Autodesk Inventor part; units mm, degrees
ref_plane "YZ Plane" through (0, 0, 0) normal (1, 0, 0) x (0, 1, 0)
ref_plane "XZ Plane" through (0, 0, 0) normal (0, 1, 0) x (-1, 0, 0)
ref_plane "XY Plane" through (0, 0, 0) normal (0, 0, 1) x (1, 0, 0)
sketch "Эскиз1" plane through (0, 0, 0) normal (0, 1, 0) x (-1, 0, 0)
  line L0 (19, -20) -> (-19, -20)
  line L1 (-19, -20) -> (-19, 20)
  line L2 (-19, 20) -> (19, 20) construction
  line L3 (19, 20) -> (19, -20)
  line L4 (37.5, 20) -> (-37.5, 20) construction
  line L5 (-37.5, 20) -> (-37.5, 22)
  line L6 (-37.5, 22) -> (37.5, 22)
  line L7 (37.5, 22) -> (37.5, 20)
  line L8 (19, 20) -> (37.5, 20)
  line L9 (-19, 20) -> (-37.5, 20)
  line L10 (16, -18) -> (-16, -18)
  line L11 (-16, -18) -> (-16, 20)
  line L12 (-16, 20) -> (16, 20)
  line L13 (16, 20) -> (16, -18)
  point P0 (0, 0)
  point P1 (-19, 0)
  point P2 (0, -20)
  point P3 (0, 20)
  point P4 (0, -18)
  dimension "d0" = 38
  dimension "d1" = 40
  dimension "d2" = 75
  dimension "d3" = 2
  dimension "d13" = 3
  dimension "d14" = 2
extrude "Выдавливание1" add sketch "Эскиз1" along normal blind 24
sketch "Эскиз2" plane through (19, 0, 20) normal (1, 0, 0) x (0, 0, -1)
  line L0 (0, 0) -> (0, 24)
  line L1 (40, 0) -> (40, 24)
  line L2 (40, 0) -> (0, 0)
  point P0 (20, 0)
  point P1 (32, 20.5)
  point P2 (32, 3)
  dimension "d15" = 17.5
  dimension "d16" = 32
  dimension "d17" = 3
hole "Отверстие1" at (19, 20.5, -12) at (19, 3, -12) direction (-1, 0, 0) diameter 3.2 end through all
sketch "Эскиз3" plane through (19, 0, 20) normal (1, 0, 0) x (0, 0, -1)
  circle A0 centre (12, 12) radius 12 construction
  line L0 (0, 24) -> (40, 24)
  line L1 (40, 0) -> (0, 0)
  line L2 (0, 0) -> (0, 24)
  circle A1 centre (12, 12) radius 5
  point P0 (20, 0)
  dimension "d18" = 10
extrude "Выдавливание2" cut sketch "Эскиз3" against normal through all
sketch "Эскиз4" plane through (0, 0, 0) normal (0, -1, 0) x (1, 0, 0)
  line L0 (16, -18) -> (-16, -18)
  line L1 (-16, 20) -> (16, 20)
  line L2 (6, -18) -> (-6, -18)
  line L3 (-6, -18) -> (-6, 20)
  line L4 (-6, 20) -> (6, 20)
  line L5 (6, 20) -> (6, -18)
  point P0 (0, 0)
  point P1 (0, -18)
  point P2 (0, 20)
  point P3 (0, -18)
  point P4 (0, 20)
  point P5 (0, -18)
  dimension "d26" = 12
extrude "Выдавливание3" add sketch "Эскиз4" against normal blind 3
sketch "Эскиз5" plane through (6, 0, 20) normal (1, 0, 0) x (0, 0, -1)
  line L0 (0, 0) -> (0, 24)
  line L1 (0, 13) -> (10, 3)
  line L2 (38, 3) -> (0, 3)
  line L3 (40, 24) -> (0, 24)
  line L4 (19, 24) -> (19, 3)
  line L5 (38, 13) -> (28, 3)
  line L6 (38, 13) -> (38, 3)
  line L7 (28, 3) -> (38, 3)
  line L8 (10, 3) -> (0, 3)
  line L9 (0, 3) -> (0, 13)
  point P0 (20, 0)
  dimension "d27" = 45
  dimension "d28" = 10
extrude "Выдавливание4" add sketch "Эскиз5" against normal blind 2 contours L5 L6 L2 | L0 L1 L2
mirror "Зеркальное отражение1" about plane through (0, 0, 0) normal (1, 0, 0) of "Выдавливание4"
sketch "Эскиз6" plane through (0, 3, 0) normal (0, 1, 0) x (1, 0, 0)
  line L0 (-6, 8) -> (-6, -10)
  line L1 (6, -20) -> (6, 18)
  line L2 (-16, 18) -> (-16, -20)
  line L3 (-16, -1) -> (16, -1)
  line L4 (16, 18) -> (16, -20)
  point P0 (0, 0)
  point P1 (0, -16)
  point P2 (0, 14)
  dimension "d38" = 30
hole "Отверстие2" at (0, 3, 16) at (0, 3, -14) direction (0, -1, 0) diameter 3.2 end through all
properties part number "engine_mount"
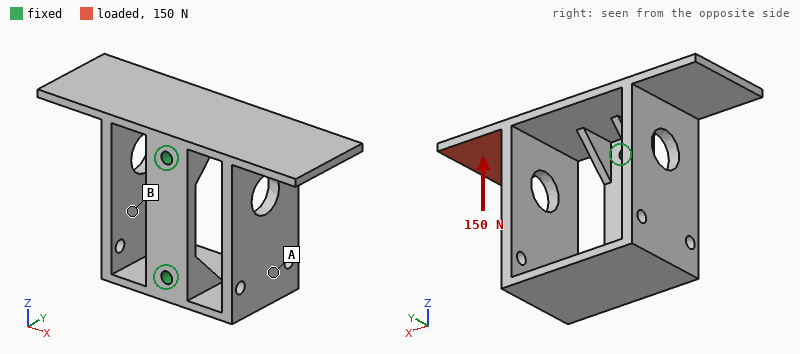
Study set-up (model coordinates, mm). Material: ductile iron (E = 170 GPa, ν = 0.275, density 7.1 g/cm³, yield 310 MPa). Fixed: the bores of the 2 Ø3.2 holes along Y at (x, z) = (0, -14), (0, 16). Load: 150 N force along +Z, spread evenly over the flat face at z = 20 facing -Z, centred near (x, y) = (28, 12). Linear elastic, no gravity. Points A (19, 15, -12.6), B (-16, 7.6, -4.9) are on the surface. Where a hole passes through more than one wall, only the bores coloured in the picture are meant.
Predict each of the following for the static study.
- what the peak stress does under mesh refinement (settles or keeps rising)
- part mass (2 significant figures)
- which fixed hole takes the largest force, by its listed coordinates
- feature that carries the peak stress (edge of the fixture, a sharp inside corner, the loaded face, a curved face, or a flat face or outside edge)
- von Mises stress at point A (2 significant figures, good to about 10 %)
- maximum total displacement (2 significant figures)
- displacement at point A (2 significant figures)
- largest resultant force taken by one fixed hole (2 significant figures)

keeps rising
86 g
(0, -14)
edge of the fixture
13 MPa
99 µm
15 µm
160 N
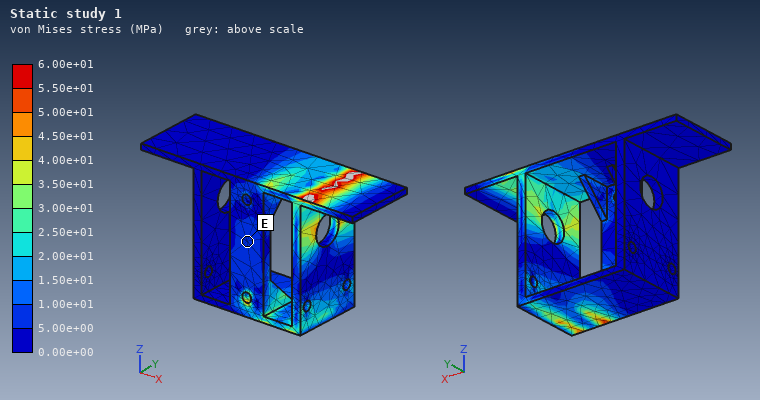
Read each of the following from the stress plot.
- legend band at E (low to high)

5.00e+00 to 1.00e+01 MPa
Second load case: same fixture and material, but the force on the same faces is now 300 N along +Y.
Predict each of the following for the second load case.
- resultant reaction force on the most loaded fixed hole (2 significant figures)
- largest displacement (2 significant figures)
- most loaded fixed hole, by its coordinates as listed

300 N
0.12 mm
(0, 16)
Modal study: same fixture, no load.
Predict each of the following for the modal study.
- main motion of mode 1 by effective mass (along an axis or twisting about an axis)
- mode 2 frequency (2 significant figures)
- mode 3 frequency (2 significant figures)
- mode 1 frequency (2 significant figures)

along X
2600 Hz
2700 Hz
1800 Hz
